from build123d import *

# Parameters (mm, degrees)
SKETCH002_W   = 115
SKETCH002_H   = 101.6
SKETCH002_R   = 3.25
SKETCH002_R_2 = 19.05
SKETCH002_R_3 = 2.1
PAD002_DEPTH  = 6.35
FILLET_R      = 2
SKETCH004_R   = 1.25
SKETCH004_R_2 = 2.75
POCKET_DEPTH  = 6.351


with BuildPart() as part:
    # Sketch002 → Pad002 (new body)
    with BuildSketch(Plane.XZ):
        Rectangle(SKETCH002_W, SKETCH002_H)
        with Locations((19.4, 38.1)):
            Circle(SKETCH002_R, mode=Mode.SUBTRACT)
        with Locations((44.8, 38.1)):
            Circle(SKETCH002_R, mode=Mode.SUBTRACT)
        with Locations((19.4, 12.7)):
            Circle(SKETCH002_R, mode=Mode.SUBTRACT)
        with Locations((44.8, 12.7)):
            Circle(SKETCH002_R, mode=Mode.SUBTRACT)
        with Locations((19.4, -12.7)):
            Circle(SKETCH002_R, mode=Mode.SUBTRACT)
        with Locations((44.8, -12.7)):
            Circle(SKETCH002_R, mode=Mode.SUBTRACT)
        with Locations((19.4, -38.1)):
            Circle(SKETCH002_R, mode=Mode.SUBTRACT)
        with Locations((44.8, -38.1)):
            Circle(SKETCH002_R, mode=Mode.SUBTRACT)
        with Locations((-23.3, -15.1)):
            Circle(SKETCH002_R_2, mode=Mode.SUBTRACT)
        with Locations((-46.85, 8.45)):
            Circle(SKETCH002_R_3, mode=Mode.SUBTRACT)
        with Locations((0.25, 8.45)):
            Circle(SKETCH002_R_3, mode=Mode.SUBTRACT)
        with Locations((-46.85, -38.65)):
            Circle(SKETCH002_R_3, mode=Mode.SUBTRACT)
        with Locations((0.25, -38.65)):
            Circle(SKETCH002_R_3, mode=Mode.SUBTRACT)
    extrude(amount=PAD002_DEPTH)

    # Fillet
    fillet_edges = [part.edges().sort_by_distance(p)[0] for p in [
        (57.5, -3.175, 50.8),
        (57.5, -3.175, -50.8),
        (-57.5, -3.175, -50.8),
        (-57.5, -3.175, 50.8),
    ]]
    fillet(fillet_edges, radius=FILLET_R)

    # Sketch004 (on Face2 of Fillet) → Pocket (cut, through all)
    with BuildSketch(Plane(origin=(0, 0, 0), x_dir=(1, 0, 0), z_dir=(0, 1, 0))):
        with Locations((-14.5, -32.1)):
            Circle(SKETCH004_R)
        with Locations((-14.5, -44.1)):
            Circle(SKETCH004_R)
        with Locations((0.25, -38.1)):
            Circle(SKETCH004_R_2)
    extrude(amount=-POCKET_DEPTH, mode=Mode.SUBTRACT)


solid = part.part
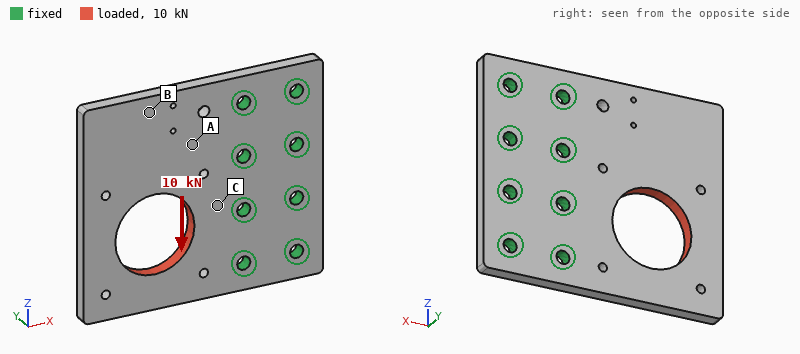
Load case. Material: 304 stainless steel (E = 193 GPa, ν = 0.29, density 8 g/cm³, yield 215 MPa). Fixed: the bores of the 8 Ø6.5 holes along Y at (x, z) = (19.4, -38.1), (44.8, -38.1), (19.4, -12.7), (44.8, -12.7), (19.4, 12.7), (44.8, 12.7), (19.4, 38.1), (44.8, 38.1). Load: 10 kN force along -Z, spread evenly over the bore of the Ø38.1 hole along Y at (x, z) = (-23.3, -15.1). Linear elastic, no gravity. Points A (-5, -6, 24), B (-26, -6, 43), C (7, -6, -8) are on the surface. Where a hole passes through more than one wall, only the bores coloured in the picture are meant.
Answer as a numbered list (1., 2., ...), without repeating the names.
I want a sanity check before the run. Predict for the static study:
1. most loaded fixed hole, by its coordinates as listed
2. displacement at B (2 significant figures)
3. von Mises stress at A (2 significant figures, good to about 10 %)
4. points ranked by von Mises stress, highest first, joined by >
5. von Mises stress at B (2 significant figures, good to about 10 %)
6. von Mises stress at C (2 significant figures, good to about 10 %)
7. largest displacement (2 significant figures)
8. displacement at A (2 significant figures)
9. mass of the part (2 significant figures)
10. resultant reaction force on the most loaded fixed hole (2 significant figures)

1. (19.4, 38.1)
2. 18 µm
3. 29 MPa
4. C > A > B
5. 15 MPa
6. 53 MPa
7. 32 µm
8. 7.2 µm
9. 520 g
10. 5.1 kN
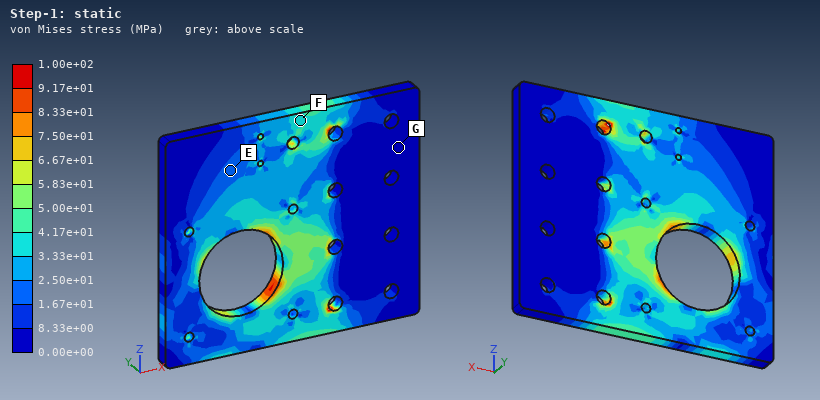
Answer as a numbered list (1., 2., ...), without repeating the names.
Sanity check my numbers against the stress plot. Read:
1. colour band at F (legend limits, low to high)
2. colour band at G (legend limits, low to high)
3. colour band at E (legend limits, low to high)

1. 3.33e+01 to 4.17e+01 MPa
2. 0.00e+00 to 8.33e+00 MPa
3. 1.67e+01 to 2.50e+01 MPa
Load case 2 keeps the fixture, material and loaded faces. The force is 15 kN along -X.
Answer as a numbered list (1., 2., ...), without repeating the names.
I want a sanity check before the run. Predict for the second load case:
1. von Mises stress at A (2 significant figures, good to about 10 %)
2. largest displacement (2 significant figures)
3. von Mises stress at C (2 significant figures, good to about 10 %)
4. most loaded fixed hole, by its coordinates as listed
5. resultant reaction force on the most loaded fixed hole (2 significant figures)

1. 20 MPa
2. 23 µm
3. 30 MPa
4. (19.4, -38.1)
5. 6.0 kN
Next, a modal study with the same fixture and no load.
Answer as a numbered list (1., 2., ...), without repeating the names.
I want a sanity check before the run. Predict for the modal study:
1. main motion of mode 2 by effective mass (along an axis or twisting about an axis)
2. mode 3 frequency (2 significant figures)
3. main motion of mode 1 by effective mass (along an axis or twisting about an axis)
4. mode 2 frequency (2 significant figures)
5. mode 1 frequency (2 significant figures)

1. twisting about X
2. 3700 Hz
3. along Y
4. 1600 Hz
5. 850 Hz
